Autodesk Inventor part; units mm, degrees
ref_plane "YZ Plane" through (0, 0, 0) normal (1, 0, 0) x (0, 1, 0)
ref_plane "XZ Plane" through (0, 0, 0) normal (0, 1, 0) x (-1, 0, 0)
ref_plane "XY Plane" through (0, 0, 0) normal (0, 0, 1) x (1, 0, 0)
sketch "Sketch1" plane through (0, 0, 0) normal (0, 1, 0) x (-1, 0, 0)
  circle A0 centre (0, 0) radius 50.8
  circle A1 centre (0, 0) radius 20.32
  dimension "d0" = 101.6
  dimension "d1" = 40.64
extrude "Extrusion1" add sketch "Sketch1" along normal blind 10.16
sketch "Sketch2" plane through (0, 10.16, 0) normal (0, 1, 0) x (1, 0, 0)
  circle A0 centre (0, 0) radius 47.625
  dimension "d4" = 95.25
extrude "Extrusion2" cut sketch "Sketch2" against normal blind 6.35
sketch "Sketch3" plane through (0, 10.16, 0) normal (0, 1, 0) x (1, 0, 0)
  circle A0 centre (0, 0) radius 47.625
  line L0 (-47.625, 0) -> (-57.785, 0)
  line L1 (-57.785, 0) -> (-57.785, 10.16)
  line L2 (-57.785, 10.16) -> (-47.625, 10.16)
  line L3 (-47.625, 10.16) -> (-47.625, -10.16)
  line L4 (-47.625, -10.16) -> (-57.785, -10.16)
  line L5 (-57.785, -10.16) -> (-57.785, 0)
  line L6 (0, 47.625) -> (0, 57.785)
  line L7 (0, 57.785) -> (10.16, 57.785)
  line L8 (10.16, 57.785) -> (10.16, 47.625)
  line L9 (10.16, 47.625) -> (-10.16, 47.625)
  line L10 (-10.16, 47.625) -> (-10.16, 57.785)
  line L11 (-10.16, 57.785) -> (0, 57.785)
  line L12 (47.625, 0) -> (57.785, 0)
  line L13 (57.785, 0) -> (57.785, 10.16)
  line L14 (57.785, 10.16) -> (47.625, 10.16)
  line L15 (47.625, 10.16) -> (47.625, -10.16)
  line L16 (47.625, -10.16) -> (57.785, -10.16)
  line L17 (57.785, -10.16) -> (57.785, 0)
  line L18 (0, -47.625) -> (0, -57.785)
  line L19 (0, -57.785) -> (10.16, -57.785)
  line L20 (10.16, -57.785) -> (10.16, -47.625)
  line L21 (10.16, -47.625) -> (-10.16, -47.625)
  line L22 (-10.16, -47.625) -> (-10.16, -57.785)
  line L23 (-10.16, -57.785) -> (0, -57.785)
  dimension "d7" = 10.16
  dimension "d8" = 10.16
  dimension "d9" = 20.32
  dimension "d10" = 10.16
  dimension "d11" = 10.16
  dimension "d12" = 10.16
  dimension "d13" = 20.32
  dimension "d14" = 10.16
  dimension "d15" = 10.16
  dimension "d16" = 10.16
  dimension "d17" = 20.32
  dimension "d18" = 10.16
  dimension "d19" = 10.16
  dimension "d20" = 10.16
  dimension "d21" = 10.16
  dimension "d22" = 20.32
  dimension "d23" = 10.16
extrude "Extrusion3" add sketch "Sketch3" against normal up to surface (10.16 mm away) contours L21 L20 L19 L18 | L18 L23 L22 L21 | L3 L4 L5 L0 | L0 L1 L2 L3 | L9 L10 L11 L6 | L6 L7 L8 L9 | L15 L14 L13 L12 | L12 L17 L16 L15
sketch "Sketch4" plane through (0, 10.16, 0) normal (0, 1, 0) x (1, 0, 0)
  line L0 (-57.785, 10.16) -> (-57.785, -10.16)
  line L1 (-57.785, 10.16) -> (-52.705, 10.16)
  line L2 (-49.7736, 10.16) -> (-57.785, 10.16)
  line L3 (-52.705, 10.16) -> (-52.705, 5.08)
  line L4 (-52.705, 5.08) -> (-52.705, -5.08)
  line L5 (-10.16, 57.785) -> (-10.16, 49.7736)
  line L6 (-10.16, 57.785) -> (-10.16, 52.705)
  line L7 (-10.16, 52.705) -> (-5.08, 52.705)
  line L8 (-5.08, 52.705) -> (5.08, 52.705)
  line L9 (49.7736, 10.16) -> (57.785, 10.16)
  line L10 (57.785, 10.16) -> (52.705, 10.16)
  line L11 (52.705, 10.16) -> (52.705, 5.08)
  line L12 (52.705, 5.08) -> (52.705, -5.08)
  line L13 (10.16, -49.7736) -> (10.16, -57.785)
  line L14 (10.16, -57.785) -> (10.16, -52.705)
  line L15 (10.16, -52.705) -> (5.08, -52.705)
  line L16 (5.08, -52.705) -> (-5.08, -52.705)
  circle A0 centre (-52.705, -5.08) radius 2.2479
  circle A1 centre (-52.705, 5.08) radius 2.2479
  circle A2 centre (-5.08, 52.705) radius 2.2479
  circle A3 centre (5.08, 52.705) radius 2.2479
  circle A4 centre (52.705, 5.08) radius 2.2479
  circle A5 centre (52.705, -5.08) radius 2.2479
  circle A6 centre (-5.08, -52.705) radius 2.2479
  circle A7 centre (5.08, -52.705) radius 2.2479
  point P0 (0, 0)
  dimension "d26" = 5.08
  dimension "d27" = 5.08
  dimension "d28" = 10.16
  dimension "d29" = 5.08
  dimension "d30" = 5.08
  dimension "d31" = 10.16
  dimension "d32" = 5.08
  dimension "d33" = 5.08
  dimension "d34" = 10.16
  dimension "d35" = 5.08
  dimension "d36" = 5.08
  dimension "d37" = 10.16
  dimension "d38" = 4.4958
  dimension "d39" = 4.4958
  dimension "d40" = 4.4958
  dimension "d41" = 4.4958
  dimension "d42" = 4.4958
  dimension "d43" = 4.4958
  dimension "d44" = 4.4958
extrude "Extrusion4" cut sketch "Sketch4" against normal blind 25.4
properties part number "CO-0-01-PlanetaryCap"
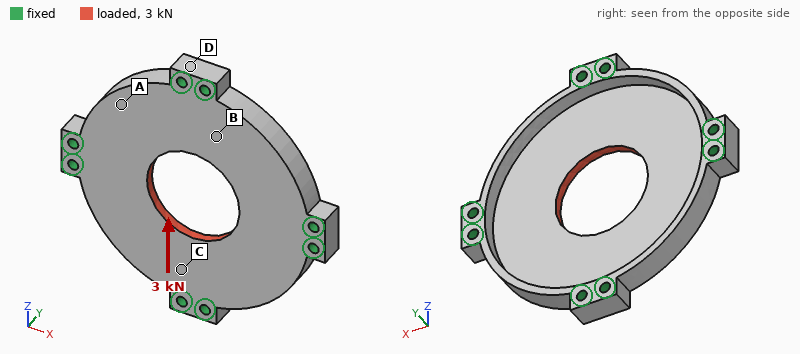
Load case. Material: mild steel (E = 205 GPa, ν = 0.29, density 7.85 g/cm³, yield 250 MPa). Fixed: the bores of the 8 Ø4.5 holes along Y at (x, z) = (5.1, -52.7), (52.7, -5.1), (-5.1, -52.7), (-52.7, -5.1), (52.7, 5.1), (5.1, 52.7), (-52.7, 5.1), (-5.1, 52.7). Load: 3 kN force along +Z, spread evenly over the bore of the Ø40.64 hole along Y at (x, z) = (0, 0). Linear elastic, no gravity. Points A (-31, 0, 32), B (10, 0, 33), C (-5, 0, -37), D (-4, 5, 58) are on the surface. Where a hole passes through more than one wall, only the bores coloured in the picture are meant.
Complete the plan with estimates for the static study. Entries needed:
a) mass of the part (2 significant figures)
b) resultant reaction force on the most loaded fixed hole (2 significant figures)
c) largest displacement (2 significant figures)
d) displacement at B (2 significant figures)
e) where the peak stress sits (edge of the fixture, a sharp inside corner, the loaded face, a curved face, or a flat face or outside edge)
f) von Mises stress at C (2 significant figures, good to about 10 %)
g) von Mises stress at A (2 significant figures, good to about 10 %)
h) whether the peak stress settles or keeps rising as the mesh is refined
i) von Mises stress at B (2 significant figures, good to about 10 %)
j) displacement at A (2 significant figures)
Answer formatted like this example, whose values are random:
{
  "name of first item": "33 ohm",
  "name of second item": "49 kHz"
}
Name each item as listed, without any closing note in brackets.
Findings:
{
  "mass of the part": "290 g",
  "resultant reaction force on the most loaded fixed hole": "490 N",
  "largest displacement": "2.0 µm",
  "displacement at B": "1.2 µm",
  "where the peak stress sits": "edge of the fixture",
  "von Mises stress at C": "10 MPa",
  "von Mises stress at A": "3.2 MPa",
  "whether the peak stress settles or keeps rising as the mesh is refined": "keeps rising",
  "von Mises stress at B": "8.7 MPa",
  "displacement at A": "1.3 µm"
}
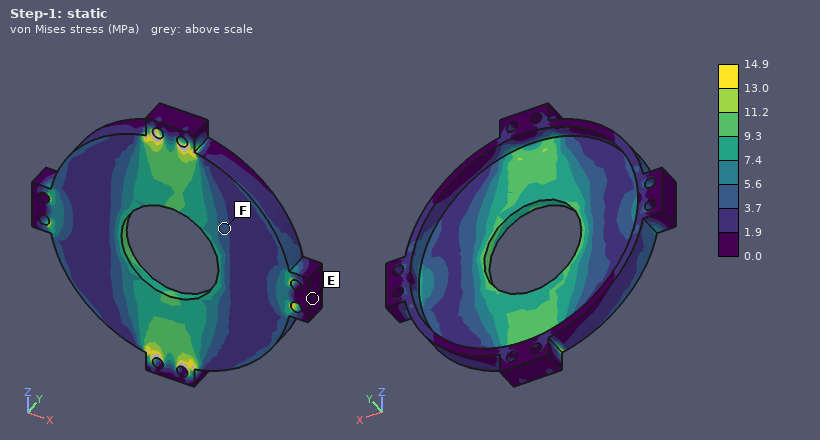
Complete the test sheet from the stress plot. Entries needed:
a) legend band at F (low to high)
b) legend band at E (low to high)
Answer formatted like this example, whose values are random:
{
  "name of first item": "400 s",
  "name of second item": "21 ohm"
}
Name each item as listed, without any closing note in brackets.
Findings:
{
  "legend band at F": "3.7 to 5.6 MPa",
  "legend band at E": "0.0 to 1.9 MPa"
}
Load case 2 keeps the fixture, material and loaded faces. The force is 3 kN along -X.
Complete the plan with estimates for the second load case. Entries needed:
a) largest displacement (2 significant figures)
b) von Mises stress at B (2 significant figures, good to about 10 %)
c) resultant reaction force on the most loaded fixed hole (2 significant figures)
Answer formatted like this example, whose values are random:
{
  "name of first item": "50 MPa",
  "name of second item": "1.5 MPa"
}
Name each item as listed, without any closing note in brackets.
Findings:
{
  "largest displacement": "2.0 µm",
  "von Mises stress at B": "2.2 MPa",
  "resultant reaction force on the most loaded fixed hole": "490 N"
}
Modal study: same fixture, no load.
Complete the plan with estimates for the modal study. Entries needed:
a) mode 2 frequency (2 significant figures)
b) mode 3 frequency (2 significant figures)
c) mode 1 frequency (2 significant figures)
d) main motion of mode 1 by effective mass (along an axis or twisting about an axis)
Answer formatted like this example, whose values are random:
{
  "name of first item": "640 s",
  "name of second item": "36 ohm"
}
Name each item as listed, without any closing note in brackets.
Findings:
{
  "mode 2 frequency": "5900 Hz",
  "mode 3 frequency": "5900 Hz",
  "mode 1 frequency": "4100 Hz",
  "main motion of mode 1 by effective mass": "along Y"
}
